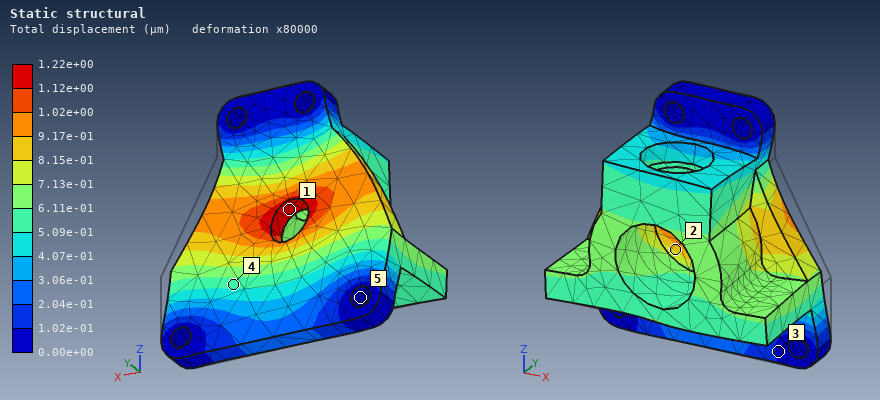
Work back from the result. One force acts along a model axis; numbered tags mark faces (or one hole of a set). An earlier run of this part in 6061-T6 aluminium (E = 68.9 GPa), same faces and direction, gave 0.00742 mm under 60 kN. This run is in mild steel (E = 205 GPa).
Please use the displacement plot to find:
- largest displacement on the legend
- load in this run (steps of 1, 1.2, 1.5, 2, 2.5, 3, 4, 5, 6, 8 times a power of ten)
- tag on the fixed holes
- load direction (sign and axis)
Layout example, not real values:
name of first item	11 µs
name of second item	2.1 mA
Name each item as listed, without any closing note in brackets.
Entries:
largest displacement on the legend	1.22e+00 µm
load in this run	30 kN
tag on the fixed holes	5
load direction	-X
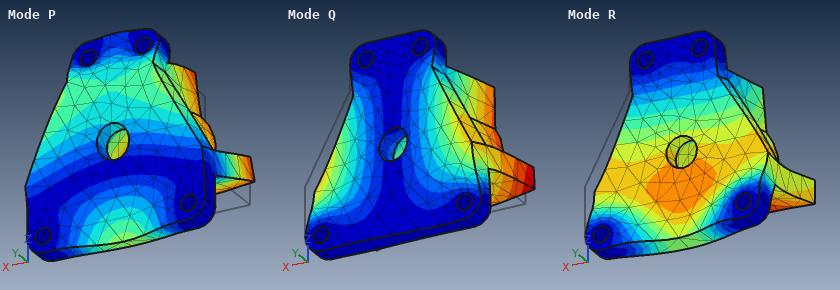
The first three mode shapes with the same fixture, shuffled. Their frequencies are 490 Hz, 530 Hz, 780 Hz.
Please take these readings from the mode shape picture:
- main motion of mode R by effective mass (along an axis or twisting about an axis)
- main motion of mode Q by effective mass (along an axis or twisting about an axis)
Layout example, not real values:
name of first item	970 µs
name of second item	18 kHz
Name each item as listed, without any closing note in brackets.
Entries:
main motion of mode R by effective mass	along Y
main motion of mode Q by effective mass	along X
